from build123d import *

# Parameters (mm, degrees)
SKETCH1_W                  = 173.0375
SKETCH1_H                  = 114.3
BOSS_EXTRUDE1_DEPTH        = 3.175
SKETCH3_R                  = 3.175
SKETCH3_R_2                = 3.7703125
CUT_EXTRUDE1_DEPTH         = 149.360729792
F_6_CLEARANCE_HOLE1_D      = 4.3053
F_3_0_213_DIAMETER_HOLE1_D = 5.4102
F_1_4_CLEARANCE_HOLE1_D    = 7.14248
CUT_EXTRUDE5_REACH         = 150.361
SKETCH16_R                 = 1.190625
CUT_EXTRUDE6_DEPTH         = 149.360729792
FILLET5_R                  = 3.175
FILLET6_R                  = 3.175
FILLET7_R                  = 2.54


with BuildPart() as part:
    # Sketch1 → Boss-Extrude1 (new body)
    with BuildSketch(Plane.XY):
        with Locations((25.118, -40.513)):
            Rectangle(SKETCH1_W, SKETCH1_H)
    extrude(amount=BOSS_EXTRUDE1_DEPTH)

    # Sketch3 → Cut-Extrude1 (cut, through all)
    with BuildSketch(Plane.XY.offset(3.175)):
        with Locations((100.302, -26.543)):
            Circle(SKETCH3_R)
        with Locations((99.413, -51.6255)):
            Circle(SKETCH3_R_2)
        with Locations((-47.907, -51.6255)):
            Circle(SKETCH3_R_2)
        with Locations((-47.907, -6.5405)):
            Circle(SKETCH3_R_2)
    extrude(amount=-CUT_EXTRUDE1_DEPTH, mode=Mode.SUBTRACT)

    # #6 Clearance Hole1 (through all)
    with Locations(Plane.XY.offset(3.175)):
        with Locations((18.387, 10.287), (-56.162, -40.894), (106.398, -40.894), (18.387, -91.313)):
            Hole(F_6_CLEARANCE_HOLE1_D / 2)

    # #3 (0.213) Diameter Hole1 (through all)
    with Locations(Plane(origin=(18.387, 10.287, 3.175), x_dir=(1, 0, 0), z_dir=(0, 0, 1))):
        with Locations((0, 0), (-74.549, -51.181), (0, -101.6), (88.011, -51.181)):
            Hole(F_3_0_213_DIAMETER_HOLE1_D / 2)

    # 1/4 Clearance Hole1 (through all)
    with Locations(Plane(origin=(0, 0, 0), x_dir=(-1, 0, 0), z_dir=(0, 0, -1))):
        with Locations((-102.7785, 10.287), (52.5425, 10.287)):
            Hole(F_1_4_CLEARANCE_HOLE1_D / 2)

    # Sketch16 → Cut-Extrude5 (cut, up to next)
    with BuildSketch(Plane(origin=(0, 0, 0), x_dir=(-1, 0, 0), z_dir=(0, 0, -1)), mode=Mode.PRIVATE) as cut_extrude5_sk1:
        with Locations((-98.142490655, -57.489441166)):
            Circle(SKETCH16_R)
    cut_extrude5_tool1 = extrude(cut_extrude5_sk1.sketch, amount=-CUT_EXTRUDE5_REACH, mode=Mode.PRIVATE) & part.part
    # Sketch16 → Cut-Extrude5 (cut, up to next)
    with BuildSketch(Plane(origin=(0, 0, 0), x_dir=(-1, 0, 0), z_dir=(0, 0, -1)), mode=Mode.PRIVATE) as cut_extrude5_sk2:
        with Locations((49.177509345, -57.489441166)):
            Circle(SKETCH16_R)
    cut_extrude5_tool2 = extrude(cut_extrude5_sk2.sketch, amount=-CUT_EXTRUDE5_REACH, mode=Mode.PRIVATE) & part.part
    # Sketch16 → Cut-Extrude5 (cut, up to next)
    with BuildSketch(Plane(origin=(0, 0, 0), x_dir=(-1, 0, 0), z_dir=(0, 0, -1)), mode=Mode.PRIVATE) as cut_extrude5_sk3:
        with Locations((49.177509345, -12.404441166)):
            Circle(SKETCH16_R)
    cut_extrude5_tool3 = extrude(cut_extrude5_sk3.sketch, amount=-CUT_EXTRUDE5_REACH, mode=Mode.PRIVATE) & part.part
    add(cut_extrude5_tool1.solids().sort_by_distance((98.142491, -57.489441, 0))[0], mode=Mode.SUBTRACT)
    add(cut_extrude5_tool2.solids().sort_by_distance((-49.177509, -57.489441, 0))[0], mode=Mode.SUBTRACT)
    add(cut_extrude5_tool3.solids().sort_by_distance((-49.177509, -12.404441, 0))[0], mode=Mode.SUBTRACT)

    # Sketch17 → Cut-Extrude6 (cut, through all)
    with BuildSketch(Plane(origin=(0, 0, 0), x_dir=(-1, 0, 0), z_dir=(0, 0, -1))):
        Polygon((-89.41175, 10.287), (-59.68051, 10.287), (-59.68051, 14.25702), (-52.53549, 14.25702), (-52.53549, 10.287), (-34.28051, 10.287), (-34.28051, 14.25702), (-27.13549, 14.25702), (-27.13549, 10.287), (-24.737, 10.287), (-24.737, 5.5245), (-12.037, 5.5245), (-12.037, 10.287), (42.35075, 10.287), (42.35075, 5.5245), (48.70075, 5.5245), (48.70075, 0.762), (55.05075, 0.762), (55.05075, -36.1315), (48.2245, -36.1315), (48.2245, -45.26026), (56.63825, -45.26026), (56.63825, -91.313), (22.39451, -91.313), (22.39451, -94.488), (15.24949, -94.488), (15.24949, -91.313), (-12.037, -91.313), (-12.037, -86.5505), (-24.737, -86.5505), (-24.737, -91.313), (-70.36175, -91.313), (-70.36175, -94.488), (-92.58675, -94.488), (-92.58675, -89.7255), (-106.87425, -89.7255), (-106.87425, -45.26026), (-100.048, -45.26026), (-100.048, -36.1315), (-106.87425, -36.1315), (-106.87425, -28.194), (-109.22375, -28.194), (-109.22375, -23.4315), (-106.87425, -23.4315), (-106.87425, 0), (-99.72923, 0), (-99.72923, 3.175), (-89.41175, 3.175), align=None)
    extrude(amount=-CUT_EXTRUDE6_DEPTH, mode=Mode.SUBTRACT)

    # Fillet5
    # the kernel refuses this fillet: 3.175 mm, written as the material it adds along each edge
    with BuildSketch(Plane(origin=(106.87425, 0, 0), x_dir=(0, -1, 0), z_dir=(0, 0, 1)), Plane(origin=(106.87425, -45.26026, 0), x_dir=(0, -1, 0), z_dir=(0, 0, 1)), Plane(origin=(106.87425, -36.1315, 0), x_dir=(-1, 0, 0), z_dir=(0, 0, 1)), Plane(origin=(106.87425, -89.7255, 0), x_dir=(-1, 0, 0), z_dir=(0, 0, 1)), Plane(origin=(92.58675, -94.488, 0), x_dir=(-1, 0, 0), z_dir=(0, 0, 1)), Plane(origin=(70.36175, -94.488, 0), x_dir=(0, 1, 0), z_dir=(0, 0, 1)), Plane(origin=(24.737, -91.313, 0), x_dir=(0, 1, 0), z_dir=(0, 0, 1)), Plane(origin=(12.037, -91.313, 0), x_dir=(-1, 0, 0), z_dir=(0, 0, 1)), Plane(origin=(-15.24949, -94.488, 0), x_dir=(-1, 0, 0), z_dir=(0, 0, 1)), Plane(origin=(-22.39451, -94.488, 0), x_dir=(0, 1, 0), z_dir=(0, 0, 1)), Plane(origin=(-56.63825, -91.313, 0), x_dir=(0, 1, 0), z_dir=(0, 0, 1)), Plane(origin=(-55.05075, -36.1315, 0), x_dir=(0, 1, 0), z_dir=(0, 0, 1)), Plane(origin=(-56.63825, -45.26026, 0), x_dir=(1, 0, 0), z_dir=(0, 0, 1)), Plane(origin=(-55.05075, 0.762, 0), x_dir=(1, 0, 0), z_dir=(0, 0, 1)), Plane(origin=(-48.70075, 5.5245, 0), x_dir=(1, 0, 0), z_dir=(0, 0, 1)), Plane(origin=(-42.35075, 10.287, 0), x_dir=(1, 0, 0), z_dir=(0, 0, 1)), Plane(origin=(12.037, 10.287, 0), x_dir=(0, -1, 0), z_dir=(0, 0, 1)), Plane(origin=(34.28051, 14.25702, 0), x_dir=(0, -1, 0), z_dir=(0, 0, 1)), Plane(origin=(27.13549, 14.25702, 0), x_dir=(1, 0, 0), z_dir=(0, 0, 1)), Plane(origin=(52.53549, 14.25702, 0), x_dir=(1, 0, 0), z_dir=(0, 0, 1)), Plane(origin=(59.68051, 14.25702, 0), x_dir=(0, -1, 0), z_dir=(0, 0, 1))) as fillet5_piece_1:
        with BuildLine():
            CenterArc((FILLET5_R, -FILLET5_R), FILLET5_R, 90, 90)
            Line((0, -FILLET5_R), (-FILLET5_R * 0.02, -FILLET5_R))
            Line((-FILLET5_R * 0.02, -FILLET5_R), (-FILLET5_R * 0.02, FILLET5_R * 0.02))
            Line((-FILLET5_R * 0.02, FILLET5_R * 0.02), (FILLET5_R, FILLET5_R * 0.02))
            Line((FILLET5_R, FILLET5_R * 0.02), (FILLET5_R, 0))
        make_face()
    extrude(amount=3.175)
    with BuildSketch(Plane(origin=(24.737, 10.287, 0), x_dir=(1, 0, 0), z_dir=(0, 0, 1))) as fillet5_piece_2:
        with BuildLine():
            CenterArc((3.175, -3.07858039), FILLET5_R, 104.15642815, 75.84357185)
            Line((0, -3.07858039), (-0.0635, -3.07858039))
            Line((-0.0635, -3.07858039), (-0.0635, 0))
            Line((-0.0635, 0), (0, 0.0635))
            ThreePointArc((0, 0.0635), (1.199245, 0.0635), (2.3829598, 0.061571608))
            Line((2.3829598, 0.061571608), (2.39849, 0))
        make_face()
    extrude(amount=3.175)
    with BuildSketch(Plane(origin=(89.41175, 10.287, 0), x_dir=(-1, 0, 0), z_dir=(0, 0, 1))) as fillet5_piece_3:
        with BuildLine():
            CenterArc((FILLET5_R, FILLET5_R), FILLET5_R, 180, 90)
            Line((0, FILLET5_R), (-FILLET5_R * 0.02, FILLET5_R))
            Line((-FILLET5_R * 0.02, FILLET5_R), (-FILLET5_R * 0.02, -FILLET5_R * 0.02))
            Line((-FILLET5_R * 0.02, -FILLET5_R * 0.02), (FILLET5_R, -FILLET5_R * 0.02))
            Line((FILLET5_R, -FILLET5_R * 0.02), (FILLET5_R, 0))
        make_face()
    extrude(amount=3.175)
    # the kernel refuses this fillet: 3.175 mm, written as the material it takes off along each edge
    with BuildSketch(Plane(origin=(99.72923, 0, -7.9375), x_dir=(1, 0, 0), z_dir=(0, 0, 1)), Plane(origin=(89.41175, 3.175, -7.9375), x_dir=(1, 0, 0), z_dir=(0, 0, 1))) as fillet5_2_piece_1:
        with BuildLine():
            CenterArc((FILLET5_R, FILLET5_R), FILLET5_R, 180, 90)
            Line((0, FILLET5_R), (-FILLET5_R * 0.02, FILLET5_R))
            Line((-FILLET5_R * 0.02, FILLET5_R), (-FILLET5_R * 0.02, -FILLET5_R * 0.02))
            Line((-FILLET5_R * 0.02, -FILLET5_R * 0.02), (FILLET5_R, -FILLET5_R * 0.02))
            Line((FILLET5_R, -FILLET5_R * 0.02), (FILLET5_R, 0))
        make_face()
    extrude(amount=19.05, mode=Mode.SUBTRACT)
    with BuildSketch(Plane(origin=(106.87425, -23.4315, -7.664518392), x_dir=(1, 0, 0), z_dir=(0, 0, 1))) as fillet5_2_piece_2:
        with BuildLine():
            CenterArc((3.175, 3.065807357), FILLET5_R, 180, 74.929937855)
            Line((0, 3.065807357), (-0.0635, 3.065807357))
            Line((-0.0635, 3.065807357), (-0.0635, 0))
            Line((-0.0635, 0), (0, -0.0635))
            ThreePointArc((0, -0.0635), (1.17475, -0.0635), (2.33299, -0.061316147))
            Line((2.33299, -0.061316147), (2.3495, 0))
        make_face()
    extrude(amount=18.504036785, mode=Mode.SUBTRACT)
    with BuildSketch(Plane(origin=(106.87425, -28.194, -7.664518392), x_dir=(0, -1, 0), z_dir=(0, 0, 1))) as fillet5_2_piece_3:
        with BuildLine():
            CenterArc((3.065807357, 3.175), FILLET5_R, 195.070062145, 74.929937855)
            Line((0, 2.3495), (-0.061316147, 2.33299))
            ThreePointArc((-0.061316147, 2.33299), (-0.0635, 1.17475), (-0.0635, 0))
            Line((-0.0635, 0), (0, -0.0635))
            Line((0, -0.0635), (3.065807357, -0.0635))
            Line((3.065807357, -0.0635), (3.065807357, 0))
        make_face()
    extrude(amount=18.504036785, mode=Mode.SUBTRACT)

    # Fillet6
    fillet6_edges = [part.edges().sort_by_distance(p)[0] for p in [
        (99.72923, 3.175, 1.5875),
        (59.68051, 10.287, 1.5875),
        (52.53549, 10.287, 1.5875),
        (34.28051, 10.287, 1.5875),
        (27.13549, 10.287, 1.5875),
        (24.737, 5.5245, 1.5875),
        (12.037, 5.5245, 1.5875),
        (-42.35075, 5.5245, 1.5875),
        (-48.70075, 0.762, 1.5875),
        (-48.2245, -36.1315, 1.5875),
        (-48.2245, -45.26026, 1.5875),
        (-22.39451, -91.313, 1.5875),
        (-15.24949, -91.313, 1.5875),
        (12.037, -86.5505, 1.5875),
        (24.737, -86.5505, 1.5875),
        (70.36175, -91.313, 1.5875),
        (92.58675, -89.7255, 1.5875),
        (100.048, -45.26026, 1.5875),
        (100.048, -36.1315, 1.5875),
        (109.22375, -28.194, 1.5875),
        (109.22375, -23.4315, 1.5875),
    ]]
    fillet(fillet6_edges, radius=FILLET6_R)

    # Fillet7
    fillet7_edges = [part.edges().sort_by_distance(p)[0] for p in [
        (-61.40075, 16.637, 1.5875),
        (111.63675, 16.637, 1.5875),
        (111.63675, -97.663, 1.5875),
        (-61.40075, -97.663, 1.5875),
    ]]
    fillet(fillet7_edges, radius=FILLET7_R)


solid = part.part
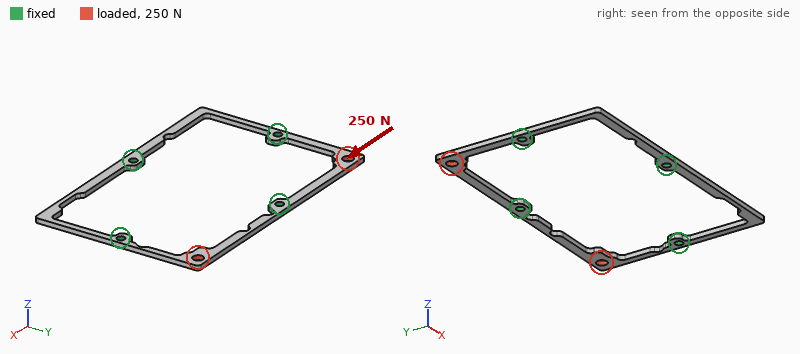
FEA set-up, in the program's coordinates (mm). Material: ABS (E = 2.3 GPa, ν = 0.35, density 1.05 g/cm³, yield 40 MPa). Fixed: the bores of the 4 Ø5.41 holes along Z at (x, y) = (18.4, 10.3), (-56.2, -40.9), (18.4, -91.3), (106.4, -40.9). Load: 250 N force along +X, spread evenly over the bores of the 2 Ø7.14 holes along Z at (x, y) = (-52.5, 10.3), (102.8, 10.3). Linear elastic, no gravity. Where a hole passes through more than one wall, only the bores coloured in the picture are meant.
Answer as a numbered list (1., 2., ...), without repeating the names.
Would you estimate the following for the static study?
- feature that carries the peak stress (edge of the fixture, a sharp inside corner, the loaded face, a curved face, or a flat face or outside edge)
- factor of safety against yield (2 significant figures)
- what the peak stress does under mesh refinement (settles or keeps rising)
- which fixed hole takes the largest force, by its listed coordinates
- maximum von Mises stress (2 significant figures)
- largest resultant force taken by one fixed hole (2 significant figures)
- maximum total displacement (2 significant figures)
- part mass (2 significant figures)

1. a curved face
2. 0.71
3. settles
4. (18.4, 10.3)
5. 56 MPa
6. 230 N
7. 0.89 mm
8. 11 g
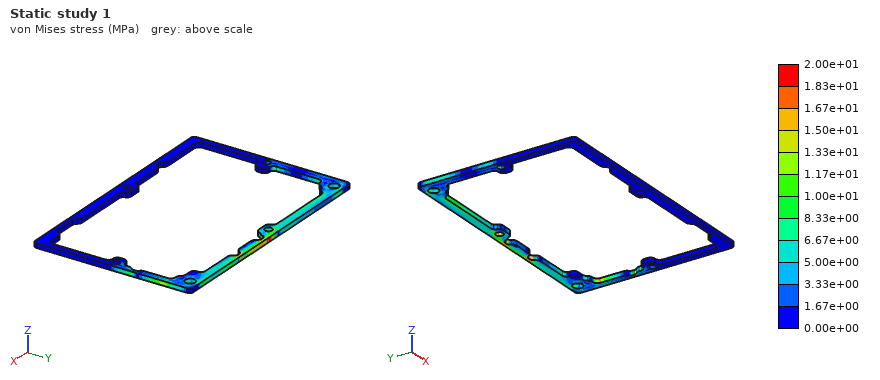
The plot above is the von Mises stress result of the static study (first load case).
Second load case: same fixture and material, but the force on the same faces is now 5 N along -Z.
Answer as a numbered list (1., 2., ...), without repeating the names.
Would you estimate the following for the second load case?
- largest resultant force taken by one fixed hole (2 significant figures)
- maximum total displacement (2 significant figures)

1. 1.8 N
2. 2.3 mm
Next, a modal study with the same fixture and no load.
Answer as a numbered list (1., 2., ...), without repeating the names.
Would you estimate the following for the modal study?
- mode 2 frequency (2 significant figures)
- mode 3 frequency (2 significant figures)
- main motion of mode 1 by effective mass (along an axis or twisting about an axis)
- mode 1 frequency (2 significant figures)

1. 210 Hz
2. 240 Hz
3. along Z
4. 170 Hz
